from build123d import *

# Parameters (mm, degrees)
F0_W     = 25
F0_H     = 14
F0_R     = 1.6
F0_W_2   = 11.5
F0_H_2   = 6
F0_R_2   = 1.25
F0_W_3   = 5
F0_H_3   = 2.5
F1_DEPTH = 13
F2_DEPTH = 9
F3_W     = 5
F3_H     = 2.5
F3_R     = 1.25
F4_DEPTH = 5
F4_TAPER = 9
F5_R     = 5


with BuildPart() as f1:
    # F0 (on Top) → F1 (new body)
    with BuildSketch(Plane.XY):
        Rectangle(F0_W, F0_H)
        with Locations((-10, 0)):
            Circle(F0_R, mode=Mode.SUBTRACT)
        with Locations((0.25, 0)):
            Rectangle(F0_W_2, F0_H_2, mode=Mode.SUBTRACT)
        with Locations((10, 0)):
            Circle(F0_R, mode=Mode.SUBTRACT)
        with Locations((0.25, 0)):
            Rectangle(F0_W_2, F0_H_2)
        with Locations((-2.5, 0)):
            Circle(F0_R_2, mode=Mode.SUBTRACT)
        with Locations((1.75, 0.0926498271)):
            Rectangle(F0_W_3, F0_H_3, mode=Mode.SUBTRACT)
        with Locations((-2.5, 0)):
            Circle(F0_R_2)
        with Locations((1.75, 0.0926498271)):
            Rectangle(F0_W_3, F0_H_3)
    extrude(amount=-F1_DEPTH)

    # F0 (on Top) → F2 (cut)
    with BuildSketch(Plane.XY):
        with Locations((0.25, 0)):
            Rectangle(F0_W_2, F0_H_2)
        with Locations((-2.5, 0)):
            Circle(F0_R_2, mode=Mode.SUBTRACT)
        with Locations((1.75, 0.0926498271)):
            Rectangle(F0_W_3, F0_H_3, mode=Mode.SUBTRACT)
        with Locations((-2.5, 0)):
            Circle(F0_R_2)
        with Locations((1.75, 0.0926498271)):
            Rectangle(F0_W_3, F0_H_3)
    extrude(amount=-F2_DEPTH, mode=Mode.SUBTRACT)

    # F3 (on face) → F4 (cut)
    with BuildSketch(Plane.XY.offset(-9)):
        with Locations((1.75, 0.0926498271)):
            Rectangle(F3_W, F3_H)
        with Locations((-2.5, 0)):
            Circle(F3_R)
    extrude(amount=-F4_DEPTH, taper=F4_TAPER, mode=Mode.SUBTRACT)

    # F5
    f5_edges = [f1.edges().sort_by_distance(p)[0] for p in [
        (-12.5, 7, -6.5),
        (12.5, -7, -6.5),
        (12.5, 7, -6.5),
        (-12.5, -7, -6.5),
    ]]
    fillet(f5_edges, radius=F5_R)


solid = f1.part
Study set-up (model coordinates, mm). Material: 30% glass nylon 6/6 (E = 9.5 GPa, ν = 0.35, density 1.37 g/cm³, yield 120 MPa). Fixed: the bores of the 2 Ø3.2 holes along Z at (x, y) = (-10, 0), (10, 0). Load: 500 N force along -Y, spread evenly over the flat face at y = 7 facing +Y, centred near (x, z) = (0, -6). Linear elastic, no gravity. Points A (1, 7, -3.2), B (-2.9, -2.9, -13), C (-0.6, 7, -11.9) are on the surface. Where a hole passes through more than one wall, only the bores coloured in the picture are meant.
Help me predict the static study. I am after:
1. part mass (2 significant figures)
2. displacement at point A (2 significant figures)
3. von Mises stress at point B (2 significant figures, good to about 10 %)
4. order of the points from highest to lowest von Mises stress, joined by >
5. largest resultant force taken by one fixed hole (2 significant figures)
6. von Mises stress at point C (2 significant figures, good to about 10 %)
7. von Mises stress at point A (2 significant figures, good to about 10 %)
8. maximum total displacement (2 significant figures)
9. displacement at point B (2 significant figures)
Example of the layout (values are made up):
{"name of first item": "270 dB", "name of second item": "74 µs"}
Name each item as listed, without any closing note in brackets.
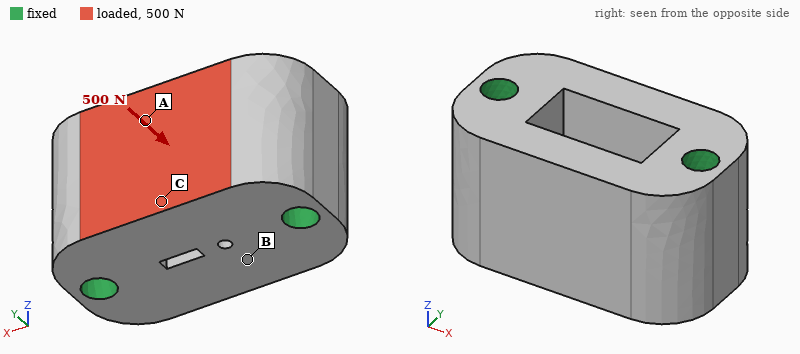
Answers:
{"part mass": "4.7 g", "displacement at point A": "12 µm", "von Mises stress at point B": "2.3 MPa", "order of the points from highest to lowest von Mises stress, joined by >": "A > C > B", "largest resultant force taken by one fixed hole": "270 N", "von Mises stress at point C": "5.3 MPa", "von Mises stress at point A": "8.7 MPa", "maximum total displacement": "16 µm", "displacement at point B": "3.8 µm"}
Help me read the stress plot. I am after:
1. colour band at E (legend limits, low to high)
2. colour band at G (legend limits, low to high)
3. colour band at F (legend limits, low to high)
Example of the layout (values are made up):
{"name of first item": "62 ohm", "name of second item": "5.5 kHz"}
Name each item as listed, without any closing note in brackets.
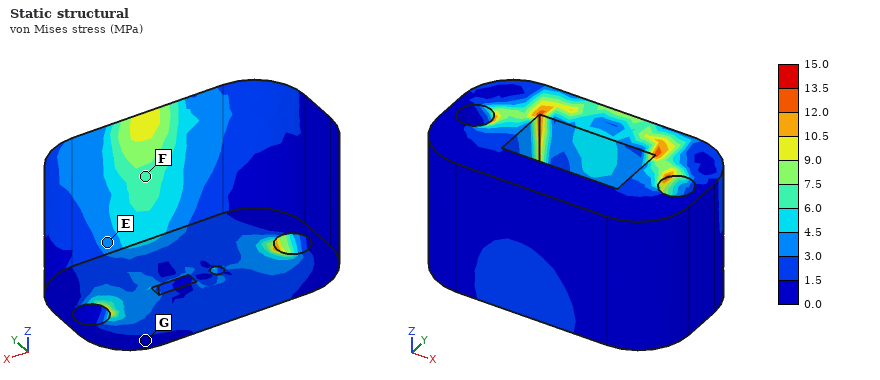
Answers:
{"colour band at E": "3.0 to 4.5 MPa", "colour band at G": "0.0 to 1.5 MPa", "colour band at F": "6.0 to 7.5 MPa"}
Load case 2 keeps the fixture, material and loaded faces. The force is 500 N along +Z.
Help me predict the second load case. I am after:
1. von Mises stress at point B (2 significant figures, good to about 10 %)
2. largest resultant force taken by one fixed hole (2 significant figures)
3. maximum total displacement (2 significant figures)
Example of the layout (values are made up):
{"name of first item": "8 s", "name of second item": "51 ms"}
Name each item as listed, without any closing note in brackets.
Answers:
{"von Mises stress at point B": "2.6 MPa", "largest resultant force taken by one fixed hole": "250 N", "maximum total displacement": "20 µm"}
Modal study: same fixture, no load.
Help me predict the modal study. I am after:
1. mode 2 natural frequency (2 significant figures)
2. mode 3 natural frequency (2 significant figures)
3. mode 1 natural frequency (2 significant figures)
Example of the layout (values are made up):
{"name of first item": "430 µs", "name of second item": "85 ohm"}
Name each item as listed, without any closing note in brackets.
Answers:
{"mode 2 natural frequency": "32 kHz", "mode 3 natural frequency": "33 kHz", "mode 1 natural frequency": "31 kHz"}
